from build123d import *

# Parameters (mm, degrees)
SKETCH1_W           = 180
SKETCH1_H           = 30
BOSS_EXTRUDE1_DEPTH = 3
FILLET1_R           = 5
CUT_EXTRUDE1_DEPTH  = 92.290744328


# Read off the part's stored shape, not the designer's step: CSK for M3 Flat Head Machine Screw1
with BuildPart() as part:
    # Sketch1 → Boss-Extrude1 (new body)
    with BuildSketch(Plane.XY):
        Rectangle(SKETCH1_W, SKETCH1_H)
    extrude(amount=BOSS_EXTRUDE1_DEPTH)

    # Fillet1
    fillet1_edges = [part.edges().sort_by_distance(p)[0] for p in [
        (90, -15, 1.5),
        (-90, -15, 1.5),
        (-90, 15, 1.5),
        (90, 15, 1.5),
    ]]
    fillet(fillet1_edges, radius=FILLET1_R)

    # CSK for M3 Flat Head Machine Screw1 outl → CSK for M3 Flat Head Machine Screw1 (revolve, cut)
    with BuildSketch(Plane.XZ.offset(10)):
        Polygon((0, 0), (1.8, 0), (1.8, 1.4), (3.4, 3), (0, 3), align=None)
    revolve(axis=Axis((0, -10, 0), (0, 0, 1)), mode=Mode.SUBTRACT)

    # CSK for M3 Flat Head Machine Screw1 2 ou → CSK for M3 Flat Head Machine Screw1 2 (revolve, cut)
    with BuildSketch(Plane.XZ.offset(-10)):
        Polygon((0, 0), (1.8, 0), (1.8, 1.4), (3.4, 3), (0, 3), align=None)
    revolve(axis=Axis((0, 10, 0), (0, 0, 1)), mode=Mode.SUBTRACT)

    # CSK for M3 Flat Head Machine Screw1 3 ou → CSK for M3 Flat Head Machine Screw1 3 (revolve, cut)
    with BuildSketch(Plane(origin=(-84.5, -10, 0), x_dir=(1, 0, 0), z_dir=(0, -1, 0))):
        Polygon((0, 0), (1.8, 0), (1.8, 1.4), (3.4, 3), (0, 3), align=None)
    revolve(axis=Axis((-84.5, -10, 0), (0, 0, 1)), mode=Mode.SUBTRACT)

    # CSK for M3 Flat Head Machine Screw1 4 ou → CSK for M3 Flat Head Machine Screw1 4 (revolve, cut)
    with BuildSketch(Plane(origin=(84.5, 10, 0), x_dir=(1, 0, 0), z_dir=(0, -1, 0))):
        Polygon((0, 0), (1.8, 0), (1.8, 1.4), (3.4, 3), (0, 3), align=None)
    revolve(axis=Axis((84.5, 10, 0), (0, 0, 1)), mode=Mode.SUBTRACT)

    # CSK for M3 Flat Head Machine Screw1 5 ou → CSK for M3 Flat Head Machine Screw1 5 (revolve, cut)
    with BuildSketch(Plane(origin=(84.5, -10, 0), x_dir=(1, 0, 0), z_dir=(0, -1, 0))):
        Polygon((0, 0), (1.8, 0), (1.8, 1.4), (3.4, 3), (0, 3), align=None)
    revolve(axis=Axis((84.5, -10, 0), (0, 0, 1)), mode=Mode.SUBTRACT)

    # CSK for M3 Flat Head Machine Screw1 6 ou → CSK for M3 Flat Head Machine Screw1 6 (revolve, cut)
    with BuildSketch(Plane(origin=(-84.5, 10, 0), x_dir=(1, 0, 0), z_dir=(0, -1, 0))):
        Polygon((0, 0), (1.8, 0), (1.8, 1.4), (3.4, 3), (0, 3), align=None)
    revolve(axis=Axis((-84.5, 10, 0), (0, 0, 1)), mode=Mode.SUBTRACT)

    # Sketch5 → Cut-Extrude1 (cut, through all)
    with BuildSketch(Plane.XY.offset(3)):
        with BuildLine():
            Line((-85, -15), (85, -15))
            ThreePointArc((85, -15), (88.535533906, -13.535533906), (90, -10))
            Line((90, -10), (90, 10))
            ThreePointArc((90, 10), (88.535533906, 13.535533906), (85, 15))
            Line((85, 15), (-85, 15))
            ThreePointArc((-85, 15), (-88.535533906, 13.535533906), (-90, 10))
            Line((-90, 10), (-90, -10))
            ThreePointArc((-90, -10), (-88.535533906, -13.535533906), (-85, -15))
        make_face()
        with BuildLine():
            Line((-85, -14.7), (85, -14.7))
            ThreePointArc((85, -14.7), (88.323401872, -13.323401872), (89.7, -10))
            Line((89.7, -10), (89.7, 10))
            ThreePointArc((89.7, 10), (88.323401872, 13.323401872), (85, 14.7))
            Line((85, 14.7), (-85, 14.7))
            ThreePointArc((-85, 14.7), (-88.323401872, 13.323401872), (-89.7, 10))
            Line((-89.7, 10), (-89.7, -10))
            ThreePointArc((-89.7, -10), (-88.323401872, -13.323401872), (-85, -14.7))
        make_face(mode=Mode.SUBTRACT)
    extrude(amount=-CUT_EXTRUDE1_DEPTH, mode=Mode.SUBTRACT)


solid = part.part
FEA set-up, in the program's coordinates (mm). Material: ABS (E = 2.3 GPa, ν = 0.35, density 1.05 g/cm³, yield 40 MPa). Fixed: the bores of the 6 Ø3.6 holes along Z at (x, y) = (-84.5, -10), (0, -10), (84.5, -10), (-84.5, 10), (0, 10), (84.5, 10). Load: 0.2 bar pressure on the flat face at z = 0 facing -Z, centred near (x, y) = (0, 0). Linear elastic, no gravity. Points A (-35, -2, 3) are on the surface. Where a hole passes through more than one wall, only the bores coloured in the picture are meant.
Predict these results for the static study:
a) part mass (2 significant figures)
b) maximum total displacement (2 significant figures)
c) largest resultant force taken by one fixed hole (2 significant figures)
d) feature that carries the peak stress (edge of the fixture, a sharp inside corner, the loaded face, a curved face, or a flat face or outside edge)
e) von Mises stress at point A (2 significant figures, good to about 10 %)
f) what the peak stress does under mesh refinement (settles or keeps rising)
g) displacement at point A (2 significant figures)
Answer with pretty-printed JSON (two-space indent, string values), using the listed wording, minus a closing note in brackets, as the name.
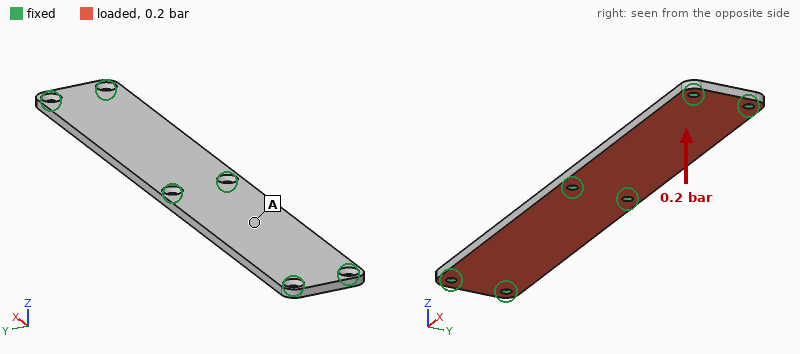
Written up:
{
  "part mass": "16 g",
  "maximum total displacement": "0.60 mm",
  "largest resultant force taken by one fixed hole": "31 N",
  "feature that carries the peak stress": "edge of the fixture",
  "von Mises stress at point A": "3.7 MPa",
  "what the peak stress does under mesh refinement": "keeps rising",
  "displacement at point A": "0.53 mm"
}
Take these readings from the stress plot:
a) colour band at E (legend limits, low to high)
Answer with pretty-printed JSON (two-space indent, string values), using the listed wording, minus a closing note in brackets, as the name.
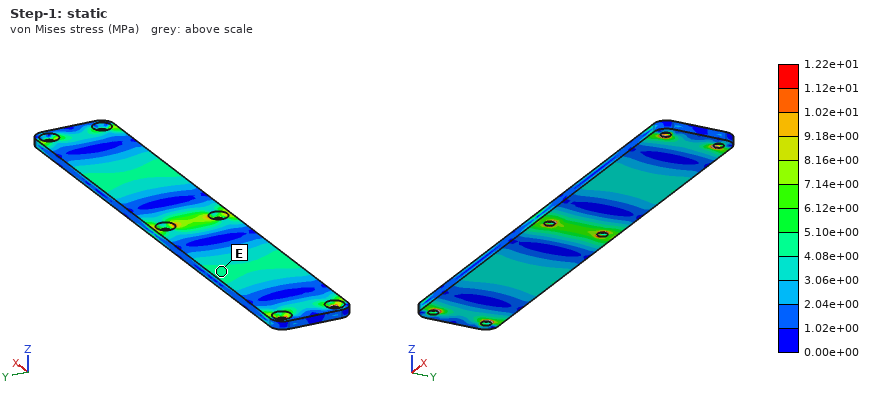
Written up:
{
  "colour band at E": "4.08e+00 to 5.10e+00 MPa"
}
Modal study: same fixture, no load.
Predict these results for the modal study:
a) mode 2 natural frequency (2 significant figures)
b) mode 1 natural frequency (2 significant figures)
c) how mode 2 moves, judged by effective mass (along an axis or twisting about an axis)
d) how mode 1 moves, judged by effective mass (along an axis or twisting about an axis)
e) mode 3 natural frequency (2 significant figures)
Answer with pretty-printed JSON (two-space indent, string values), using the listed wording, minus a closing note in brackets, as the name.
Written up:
{
  "mode 2 natural frequency": "600 Hz",
  "mode 1 natural frequency": "560 Hz",
  "how mode 2 moves, judged by effective mass": "along Z",
  "how mode 1 moves, judged by effective mass": "twisting about Y",
  "mode 3 natural frequency": "1200 Hz"
}
